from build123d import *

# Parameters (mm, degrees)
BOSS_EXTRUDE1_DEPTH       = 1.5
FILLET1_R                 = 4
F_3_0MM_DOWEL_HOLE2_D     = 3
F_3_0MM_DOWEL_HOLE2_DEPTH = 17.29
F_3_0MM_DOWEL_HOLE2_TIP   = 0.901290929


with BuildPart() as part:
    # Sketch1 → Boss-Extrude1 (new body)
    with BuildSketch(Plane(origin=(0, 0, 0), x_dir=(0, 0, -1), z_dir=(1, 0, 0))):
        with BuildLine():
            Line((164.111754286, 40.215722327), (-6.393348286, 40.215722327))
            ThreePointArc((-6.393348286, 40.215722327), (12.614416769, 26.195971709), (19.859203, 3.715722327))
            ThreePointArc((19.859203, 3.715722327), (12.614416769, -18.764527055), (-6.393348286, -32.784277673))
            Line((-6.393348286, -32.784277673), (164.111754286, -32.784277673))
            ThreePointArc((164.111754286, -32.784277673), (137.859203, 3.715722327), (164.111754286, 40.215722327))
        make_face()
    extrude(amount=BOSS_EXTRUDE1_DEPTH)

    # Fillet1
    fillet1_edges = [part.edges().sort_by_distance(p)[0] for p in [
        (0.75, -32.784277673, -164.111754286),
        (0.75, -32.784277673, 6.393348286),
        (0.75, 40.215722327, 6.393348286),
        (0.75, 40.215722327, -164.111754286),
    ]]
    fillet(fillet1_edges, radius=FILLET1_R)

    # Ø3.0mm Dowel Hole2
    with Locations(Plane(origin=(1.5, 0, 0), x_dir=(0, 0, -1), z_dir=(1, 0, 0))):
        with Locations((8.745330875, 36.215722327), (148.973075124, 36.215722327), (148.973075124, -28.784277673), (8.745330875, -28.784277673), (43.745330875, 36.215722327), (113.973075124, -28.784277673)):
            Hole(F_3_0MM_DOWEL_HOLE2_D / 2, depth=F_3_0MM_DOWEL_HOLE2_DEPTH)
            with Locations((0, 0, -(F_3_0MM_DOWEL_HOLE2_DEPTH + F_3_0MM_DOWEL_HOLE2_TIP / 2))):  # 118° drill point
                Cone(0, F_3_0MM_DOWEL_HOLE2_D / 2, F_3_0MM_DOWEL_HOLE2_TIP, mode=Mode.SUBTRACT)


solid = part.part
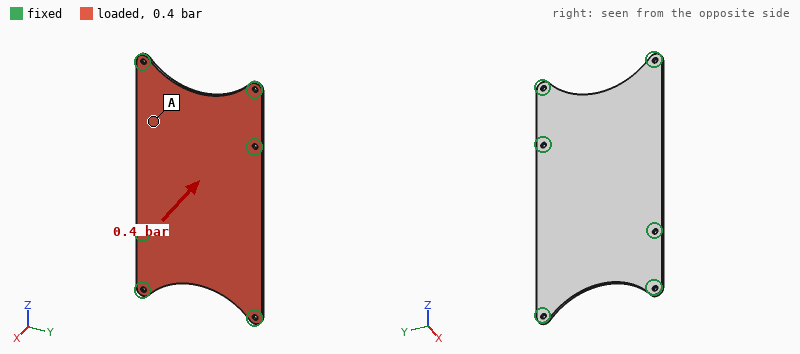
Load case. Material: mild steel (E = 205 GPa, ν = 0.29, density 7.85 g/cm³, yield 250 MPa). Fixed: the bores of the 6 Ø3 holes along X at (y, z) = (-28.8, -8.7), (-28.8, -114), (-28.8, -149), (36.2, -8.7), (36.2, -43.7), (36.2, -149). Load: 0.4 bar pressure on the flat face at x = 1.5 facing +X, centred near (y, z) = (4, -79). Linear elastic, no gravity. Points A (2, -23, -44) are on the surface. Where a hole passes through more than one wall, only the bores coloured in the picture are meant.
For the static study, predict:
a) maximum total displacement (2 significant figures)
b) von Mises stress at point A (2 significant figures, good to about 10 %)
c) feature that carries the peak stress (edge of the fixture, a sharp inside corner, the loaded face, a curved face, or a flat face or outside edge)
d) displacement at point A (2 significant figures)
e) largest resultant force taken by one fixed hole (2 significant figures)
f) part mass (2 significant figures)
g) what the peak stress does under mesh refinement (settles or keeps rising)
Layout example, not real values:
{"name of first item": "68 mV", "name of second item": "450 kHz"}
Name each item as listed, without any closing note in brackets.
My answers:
{"maximum total displacement": "0.25 mm", "von Mises stress at point A": "32 MPa", "feature that carries the peak stress": "edge of the fixture", "displacement at point A": "0.20 mm", "largest resultant force taken by one fixed hole": "130 N", "part mass": "110 g", "what the peak stress does under mesh refinement": "keeps rising"}
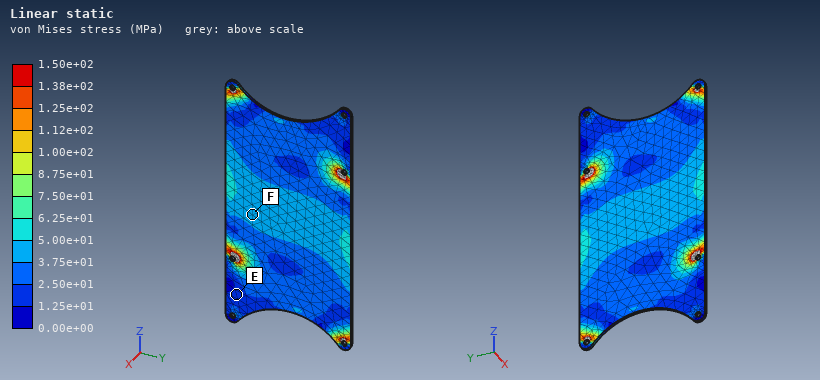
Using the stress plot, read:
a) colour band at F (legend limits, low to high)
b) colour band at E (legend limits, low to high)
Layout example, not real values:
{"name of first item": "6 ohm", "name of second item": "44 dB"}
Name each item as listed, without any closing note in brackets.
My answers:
{"colour band at F": "3.75e+01 to 5.00e+01 MPa", "colour band at E": "1.25e+01 to 2.50e+01 MPa"}
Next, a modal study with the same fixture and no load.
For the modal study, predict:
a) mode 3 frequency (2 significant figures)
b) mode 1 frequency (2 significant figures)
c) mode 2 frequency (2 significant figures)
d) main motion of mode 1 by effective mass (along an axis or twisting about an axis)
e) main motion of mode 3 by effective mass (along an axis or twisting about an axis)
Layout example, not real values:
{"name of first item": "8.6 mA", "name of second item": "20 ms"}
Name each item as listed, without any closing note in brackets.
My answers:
{"mode 3 frequency": "1700 Hz", "mode 1 frequency": "680 Hz", "mode 2 frequency": "830 Hz", "main motion of mode 1 by effective mass": "along X", "main motion of mode 3 by effective mass": "twisting about Y"}
